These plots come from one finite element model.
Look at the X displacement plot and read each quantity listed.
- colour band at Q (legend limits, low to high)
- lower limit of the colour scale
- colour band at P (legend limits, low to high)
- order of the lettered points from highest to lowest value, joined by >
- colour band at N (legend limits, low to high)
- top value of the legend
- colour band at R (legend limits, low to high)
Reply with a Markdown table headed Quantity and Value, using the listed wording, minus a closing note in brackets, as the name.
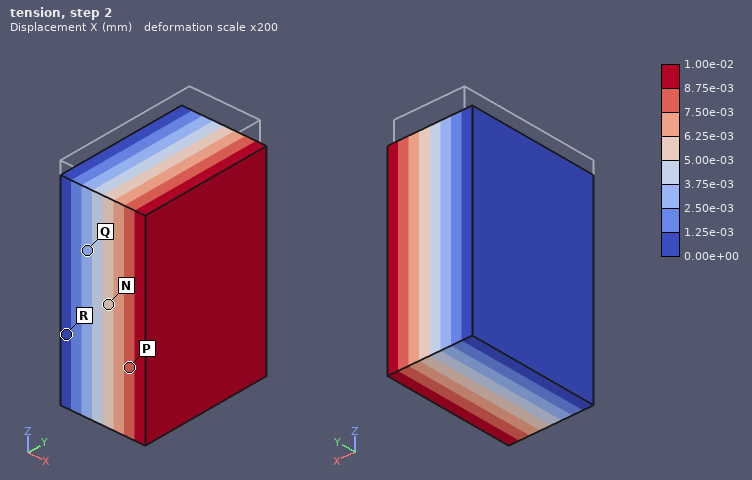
| Quantity | Value |
|---|---|
| colour band at Q | 2.50e-03 to 3.75e-03 mm |
| lower limit of the colour scale | 0.00e+00 mm |
| colour band at P | 7.50e-03 to 8.75e-03 mm |
| order of the lettered points from highest to lowest value, joined by > | P > N > Q > R |
| colour band at N | 5.00e-03 to 6.25e-03 mm |
| top value of the legend | 1.00e-02 mm |
| colour band at R | 0.00e+00 to 1.25e-03 mm |
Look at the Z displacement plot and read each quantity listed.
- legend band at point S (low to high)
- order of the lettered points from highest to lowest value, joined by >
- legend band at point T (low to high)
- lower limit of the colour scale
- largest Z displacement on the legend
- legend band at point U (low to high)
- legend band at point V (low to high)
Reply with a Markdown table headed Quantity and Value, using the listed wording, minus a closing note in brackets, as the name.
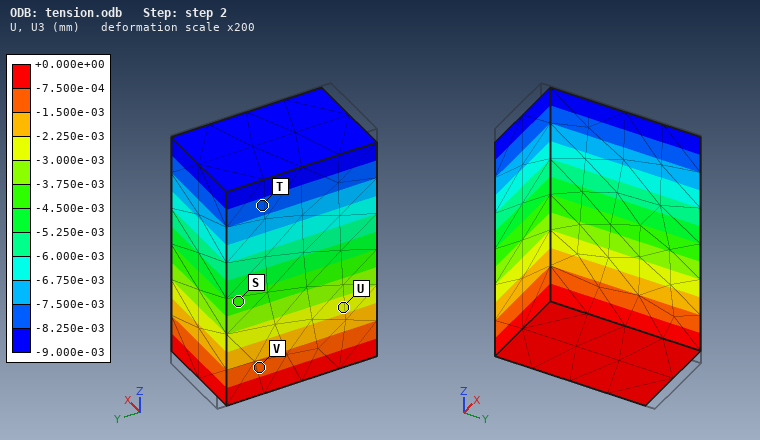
| Quantity | Value |
|---|---|
| legend band at point S | -4.500e-03 to -3.750e-03 mm |
| order of the lettered points from highest to lowest value, joined by > | V > U > S > T |
| legend band at point T | -8.250e-03 to -7.500e-03 mm |
| lower limit of the colour scale | -9.000e-03 mm |
| largest Z displacement on the legend | +0.000e+00 mm |
| legend band at point U | -3.000e-03 to -2.250e-03 mm |
| legend band at point V | -1.500e-03 to -7.500e-04 mm |
